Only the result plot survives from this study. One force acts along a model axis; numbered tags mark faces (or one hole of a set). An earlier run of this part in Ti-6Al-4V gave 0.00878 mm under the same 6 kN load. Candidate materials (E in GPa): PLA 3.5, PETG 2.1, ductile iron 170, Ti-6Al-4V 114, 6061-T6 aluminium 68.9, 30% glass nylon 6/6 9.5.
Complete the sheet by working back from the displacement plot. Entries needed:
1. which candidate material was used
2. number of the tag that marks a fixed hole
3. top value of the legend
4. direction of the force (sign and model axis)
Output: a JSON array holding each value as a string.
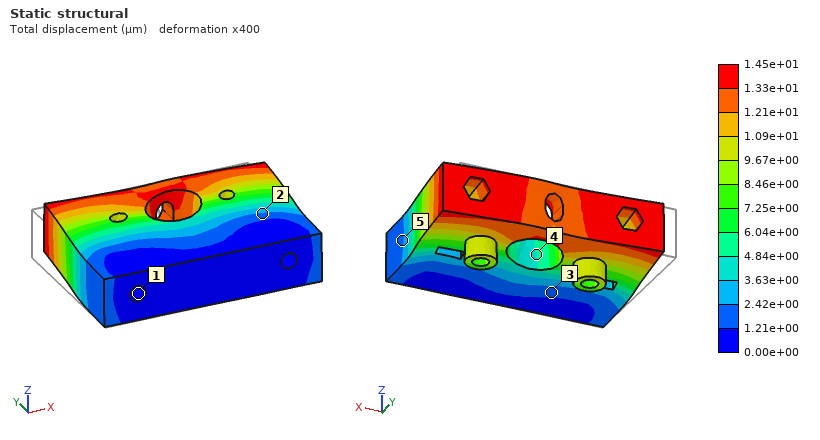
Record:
["6061-T6 aluminium", "1", "1.45e+01 µm", "+X"]
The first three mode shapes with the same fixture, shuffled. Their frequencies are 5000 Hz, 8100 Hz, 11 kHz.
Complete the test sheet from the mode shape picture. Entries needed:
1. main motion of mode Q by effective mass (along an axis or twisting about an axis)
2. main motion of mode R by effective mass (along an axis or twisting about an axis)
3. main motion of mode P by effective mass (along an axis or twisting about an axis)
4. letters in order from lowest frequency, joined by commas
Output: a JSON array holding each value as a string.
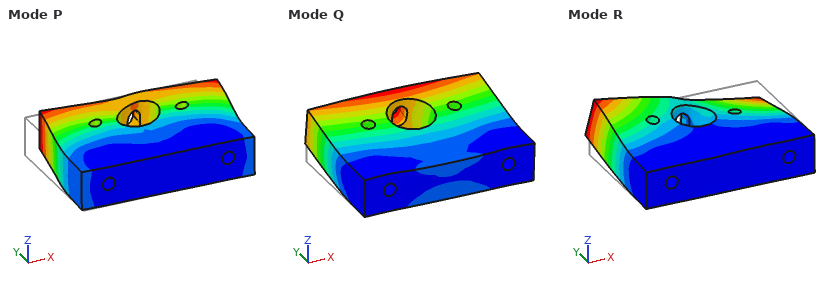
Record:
["along Z", "twisting about Y", "along X", "Q, R, P"]
